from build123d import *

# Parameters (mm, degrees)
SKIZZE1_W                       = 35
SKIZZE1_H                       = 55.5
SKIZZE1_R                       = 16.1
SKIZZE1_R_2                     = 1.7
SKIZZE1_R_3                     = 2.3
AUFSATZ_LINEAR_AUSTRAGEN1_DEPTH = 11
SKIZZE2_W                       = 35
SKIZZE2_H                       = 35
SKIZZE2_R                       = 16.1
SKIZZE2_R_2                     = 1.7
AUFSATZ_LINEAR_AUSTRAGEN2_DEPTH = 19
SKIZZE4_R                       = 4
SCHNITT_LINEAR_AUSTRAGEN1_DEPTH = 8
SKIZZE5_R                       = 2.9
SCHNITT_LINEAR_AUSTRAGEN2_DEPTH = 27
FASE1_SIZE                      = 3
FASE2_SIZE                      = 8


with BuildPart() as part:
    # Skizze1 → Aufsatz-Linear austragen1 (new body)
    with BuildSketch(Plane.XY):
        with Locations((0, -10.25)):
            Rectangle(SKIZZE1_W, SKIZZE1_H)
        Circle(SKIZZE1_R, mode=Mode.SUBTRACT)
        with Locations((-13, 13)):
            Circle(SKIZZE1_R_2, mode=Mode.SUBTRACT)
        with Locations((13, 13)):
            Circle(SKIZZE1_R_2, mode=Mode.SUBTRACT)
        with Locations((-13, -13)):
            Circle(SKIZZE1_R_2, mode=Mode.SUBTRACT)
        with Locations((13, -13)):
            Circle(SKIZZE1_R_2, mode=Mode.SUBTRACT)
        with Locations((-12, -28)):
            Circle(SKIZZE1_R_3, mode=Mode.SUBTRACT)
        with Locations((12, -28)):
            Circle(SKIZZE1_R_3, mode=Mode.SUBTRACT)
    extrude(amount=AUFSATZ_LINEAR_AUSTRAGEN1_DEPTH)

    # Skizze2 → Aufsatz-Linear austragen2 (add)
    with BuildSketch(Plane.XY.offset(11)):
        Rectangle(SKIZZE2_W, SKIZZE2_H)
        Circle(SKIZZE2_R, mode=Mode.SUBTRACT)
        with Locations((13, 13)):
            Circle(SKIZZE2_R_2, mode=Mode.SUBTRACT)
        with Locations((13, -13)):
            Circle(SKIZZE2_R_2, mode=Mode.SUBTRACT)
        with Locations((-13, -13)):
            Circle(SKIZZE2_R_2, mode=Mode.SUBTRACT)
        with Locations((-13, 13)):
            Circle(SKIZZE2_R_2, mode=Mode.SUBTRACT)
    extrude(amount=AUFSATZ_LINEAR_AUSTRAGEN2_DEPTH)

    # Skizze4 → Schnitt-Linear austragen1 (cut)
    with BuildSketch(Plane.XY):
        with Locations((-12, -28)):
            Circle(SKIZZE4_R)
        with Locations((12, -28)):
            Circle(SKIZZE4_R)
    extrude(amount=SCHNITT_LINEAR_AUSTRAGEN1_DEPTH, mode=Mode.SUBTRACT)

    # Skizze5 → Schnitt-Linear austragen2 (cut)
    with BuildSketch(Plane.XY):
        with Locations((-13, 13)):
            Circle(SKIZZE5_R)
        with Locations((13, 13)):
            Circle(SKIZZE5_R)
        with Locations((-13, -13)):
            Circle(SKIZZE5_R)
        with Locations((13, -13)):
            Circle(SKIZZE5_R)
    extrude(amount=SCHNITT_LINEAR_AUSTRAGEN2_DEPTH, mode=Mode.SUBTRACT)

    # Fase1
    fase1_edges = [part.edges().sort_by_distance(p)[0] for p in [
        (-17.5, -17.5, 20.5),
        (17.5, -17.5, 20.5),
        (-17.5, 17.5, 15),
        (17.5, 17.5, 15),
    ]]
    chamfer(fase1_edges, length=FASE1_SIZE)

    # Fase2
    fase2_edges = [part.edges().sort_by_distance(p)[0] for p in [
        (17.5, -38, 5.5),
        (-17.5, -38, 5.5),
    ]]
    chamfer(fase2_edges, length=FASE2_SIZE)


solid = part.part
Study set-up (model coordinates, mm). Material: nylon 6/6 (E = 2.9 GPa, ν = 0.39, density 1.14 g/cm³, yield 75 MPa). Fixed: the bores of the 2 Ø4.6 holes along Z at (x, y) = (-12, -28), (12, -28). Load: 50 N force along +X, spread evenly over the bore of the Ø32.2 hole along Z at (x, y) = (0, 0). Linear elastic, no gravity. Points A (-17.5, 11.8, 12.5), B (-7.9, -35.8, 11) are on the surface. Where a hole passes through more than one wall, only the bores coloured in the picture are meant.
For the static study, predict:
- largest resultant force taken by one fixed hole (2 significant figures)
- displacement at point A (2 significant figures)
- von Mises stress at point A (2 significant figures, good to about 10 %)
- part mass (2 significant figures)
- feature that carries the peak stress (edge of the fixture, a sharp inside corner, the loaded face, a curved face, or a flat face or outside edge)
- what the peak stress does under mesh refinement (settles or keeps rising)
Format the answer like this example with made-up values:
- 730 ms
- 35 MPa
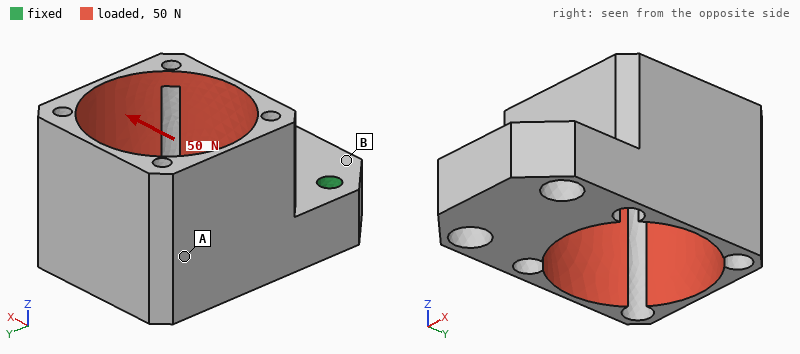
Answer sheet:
- 59 N
- 0.59 mm
- 3.3 MPa
- 18 g
- a sharp inside corner
- keeps rising
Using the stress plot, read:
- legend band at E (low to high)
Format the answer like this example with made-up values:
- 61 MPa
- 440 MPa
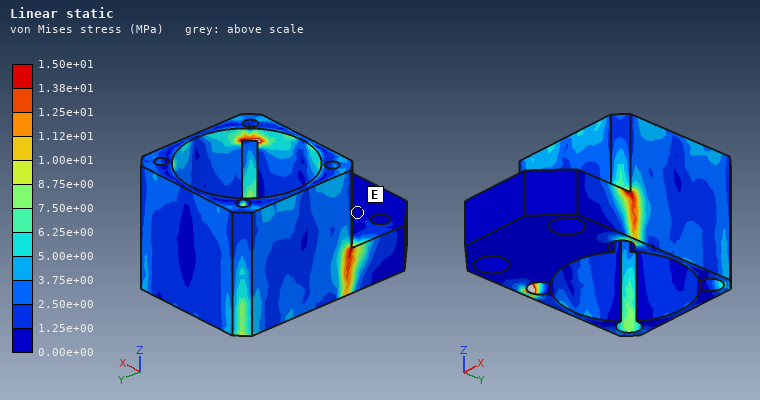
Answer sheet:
- 0.00e+00 to 1.25e+00 MPa
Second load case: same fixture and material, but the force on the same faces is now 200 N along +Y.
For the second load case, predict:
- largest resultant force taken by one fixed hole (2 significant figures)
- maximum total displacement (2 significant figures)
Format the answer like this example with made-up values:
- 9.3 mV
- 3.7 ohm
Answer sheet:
- 100 N
- 0.82 mm
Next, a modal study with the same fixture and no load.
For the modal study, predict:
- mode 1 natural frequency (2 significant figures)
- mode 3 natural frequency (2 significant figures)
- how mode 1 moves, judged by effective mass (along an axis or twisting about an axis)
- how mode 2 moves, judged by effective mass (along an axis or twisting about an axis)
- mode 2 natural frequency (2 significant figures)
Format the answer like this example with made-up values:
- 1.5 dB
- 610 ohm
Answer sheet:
- 470 Hz
- 1200 Hz
- along X
- along Z
- 550 Hz
